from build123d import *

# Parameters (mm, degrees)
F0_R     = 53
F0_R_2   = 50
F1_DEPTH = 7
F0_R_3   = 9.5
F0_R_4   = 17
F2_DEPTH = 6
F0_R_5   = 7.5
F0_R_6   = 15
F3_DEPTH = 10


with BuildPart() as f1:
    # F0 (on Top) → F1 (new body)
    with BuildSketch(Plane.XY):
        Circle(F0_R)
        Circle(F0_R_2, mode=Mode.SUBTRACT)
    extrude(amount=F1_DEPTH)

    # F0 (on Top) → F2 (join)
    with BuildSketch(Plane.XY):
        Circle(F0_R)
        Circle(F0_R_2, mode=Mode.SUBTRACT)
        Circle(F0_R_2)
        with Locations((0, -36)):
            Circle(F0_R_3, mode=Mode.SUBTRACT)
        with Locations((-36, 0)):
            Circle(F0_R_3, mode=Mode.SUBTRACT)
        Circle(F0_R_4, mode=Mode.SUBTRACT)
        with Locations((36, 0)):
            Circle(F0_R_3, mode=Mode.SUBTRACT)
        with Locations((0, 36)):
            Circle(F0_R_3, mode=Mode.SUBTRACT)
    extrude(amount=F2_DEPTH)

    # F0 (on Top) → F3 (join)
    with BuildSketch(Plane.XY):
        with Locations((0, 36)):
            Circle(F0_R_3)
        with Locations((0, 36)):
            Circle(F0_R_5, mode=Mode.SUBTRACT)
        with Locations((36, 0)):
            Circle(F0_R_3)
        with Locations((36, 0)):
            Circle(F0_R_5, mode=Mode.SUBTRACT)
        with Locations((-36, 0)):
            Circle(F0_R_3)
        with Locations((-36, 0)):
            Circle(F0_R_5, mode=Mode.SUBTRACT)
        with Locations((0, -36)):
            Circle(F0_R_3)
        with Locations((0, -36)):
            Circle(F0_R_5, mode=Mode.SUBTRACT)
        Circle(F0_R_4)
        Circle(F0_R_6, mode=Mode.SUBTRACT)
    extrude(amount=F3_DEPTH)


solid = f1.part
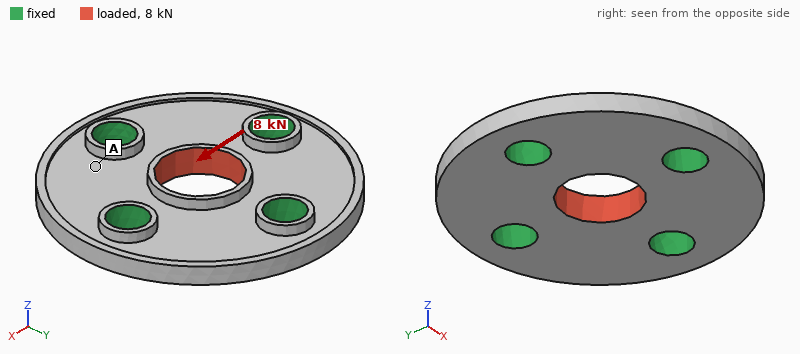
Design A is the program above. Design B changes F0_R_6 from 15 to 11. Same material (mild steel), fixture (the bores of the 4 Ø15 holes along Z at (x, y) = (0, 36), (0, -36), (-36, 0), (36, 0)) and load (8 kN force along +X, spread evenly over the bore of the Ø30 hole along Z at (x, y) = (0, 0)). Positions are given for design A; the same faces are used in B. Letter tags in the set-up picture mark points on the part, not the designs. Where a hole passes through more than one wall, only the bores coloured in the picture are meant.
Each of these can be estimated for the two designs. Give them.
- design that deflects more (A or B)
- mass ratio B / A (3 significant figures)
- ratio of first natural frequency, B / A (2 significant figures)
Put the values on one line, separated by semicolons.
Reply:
A; 1.07; 1.0
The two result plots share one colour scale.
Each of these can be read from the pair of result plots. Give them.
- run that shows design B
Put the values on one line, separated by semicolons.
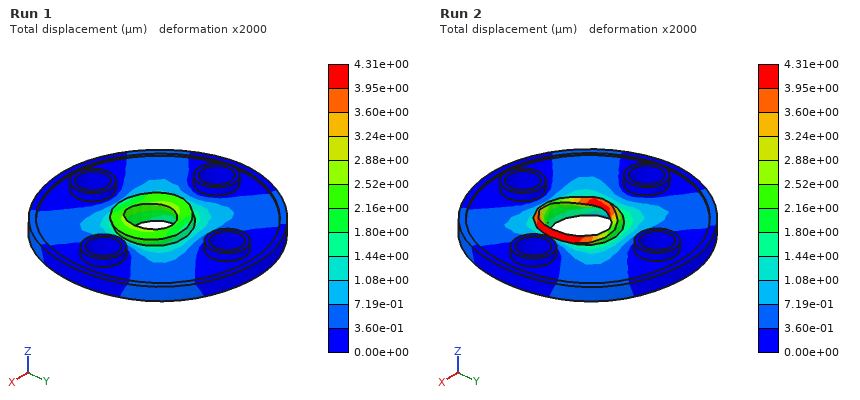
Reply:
Run 1
